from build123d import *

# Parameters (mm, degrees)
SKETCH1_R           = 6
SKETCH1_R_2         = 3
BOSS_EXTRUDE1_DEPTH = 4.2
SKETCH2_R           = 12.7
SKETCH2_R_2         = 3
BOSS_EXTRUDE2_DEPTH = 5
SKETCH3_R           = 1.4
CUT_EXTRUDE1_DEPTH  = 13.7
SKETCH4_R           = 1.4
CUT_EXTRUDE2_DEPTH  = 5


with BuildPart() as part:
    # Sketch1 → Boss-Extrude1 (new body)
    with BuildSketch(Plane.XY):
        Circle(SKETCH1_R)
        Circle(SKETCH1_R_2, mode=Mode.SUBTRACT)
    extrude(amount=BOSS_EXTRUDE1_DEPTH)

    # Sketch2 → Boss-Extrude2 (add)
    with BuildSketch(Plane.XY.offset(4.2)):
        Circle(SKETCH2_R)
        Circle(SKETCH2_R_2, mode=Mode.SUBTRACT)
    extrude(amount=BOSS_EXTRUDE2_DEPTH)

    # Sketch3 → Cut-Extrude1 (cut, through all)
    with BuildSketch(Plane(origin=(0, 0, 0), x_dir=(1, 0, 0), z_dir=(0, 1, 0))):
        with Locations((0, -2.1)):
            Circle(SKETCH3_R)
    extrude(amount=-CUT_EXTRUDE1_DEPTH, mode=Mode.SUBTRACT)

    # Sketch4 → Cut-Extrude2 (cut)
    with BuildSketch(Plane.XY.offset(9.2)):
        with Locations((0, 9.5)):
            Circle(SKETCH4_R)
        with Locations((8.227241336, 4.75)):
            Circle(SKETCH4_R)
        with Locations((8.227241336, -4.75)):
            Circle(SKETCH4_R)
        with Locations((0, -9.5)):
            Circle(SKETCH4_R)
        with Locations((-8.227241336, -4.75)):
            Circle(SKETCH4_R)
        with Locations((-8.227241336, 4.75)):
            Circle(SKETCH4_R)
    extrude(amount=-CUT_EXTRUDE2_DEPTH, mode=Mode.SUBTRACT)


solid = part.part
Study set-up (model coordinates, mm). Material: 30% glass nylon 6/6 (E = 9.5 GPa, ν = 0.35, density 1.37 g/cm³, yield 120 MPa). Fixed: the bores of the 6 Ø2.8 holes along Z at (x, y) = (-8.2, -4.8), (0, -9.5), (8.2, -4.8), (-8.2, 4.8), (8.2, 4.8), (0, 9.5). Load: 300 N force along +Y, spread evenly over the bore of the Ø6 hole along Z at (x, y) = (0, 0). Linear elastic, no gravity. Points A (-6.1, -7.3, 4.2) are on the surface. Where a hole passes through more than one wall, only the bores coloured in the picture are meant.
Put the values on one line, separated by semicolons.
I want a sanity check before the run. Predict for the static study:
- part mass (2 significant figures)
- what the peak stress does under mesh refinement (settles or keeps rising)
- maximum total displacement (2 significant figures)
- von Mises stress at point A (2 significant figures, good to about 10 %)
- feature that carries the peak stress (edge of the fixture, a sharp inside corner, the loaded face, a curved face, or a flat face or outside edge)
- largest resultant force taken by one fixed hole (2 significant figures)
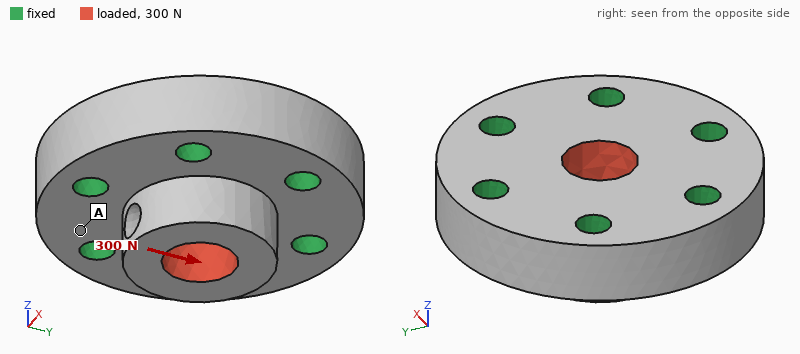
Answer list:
3.5 g; keeps rising; 4.8 µm; 0.82 MPa; a sharp inside corner; 83 N
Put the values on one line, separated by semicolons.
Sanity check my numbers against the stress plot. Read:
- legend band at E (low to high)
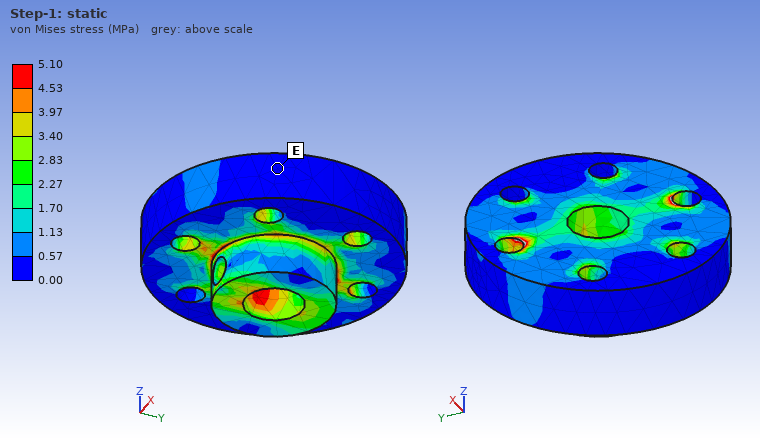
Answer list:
0.00 to 0.57 MPa
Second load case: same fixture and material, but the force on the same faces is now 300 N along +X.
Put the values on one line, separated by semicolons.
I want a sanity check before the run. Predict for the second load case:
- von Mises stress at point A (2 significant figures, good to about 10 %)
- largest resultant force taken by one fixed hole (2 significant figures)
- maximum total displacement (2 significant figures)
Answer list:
0.57 MPa; 74 N; 5.1 µm
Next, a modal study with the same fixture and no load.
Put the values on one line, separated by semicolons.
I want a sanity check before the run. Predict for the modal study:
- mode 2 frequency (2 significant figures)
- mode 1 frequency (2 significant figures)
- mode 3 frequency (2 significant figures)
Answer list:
48 kHz; 47 kHz; 49 kHz
